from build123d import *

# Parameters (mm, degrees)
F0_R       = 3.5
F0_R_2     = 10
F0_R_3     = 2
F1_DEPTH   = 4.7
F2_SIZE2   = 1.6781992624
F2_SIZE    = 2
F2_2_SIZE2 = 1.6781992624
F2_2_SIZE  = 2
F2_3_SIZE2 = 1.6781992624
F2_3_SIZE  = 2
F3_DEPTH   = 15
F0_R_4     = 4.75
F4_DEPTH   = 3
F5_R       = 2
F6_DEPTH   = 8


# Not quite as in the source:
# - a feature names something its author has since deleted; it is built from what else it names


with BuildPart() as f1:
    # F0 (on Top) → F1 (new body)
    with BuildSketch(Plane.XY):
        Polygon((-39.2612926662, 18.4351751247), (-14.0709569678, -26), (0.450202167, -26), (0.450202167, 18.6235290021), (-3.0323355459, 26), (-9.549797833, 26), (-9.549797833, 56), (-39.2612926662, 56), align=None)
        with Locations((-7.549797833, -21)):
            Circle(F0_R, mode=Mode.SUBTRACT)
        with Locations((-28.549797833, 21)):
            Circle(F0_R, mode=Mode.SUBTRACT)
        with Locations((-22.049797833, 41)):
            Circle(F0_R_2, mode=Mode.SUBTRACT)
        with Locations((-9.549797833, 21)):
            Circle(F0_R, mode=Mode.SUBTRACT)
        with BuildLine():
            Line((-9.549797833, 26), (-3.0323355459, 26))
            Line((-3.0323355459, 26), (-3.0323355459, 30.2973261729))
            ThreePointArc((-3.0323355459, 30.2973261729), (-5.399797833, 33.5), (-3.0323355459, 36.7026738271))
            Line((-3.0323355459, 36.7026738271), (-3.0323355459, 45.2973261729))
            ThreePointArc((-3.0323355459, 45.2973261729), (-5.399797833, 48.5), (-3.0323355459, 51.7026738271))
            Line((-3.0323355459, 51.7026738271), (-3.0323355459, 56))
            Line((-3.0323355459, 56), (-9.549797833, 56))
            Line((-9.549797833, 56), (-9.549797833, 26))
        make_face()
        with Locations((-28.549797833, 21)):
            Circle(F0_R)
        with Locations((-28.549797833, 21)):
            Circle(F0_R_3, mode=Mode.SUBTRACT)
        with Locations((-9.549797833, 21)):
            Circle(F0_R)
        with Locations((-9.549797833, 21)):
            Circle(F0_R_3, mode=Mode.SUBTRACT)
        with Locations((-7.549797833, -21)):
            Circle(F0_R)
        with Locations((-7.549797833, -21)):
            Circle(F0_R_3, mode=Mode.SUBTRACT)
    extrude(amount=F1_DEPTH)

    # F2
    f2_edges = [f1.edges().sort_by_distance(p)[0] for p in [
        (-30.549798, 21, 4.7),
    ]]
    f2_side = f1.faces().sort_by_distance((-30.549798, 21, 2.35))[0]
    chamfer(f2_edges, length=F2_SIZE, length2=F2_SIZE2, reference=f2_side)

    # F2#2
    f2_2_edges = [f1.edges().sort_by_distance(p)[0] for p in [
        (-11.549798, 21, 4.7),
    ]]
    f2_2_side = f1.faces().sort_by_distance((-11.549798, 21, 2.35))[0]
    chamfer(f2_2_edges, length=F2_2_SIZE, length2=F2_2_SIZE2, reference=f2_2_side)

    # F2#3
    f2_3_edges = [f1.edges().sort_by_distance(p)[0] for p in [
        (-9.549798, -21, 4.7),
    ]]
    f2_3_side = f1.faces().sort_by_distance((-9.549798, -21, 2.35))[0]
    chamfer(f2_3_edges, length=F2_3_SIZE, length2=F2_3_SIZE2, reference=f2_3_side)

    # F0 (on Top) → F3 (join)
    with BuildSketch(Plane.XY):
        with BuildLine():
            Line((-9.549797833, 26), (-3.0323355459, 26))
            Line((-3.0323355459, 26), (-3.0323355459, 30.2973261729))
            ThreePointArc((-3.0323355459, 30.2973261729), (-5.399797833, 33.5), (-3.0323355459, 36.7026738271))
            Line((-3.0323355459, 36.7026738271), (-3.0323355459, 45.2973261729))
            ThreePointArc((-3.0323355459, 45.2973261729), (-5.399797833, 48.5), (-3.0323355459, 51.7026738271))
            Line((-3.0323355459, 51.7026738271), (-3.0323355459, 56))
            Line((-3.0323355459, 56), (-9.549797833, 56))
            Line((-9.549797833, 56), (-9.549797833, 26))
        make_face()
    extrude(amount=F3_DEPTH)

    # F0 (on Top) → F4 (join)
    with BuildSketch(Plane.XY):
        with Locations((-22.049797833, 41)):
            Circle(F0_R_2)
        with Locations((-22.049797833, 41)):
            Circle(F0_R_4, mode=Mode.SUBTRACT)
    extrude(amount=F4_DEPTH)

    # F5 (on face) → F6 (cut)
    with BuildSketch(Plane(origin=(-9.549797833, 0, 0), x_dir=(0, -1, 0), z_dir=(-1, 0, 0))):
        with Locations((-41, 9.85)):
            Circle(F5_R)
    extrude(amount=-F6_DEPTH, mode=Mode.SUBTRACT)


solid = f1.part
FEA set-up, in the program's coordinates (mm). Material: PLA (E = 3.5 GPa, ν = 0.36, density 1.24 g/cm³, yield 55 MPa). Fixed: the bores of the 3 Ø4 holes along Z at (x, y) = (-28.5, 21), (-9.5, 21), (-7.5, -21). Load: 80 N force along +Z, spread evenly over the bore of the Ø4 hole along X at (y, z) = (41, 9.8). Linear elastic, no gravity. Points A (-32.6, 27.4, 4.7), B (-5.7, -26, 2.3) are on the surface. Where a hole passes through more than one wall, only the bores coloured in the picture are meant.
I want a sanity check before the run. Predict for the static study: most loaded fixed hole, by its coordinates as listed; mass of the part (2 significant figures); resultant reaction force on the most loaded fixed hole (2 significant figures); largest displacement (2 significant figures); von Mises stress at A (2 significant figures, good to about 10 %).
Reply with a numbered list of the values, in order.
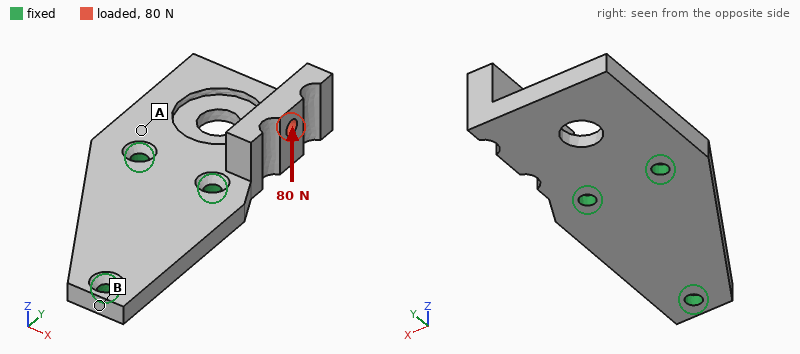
1. (-9.5, 21)
2. 16 g
3. 97 N
4. 0.79 mm
5. 5.4 MPa
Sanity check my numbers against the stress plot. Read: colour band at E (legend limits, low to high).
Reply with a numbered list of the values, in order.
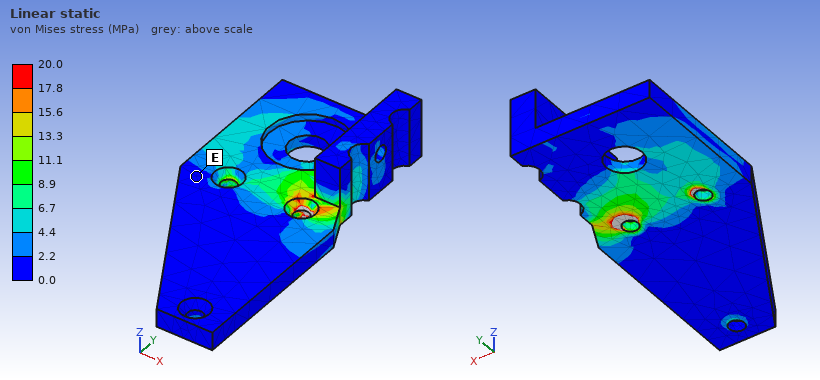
1. 0.0 to 2.2 MPa
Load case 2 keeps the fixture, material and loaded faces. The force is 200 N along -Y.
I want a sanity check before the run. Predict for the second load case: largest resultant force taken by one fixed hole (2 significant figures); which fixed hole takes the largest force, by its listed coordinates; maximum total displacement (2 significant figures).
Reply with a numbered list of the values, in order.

1. 170 N
2. (-9.5, 21)
3. 0.89 mm
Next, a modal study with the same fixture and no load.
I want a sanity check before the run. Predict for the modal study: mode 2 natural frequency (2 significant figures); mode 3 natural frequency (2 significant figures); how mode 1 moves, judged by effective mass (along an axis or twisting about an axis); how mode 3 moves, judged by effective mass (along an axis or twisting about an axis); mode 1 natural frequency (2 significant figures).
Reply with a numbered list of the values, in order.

1. 1600 Hz
2. 3100 Hz
3. along Z
4. along X
5. 830 Hz
